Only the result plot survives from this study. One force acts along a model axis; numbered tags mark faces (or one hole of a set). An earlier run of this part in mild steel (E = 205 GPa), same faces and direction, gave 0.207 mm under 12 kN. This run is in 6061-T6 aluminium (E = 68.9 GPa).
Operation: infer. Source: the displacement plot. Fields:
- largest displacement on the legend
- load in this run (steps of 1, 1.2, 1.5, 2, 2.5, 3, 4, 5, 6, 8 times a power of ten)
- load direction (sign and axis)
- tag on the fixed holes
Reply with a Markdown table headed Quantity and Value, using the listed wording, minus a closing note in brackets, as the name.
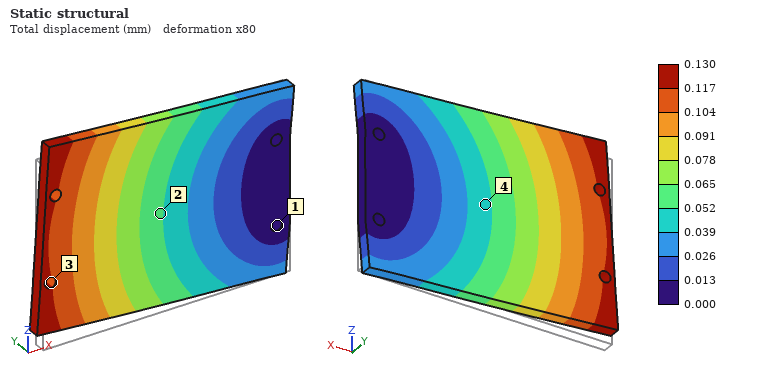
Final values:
| Quantity | Value |
|---|---|
| largest displacement on the legend | 0.130 mm |
| load in this run | 2.5 kN |
| load direction | +Z |
| tag on the fixed holes | 1 |
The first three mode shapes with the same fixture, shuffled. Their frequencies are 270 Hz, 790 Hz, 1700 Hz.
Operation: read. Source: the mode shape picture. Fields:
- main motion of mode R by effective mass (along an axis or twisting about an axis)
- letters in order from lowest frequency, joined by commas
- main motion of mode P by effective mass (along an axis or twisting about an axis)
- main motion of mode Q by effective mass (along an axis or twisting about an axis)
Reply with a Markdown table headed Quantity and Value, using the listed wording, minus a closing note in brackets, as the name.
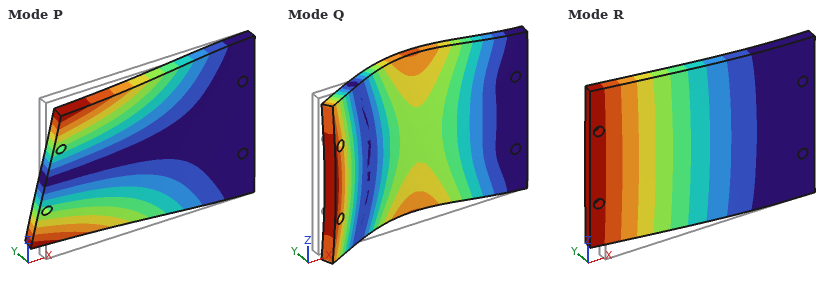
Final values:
| Quantity | Value |
|---|---|
| main motion of mode R by effective mass | along Y |
| letters in order from lowest frequency, joined by commas | R, P, Q |
| main motion of mode P by effective mass | twisting about X |
| main motion of mode Q by effective mass | along Y |
